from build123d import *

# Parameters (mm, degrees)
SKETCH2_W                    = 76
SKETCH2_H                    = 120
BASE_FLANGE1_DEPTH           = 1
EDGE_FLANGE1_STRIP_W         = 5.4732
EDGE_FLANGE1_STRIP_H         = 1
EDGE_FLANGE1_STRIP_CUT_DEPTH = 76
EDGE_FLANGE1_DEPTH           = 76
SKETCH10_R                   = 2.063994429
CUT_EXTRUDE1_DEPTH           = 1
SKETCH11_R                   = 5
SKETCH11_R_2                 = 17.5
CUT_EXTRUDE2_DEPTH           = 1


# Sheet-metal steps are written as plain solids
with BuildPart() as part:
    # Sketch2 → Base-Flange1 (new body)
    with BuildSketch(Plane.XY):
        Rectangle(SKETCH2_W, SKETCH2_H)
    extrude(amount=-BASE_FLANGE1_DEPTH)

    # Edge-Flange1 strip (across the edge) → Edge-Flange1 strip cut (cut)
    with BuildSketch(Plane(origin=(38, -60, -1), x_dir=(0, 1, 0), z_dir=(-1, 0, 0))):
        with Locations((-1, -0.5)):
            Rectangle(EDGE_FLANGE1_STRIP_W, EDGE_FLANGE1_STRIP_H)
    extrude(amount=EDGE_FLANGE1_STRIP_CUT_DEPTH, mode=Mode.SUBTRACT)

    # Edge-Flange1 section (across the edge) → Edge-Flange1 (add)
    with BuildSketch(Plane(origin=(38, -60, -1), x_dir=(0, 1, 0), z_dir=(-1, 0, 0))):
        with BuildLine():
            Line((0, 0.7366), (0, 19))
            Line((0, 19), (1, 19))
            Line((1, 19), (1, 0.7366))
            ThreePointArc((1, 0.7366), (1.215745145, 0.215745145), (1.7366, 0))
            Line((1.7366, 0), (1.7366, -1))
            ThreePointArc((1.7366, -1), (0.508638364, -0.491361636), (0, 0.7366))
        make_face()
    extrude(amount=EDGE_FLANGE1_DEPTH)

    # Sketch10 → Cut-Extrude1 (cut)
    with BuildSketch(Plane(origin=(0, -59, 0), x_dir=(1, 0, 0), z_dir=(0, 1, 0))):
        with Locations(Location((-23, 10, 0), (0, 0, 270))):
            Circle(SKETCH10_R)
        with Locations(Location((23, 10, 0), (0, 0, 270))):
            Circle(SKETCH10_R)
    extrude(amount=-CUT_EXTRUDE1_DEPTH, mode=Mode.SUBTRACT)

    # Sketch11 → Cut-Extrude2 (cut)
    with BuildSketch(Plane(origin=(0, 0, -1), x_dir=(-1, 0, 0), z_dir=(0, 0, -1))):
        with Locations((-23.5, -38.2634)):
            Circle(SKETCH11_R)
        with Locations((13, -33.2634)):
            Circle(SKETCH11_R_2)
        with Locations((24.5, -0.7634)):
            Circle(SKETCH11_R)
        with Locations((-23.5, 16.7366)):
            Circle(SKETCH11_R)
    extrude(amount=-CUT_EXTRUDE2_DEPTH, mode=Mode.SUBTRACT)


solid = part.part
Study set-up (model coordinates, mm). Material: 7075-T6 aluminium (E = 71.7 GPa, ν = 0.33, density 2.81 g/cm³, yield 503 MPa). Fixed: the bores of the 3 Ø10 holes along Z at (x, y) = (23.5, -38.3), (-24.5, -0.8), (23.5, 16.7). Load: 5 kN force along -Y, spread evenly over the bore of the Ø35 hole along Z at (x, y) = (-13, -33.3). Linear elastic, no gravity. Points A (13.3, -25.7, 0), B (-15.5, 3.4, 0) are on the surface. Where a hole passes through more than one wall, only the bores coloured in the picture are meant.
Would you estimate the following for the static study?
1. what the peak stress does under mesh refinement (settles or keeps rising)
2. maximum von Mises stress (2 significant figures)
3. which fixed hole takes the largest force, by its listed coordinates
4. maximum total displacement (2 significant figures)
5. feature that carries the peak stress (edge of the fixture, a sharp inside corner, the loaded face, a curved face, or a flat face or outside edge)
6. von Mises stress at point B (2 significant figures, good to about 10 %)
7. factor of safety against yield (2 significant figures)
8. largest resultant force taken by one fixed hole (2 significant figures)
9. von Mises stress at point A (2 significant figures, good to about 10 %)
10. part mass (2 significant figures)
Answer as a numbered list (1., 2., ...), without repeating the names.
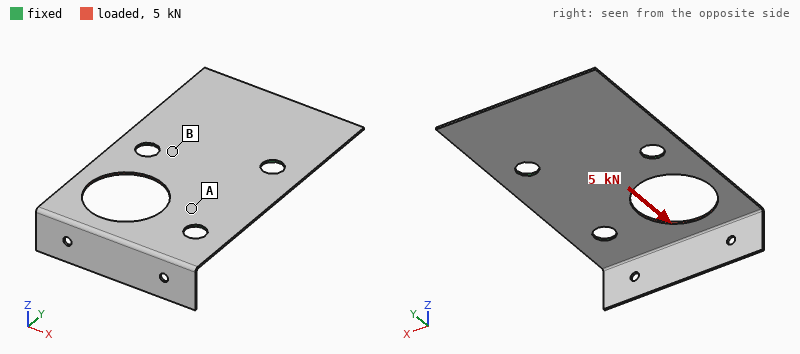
1. settles
2. 360 MPa
3. (-24.5, -0.8)
4. 0.17 mm
5. the loaded face
6. 28 MPa
7. 1.4
8. 2.9 kN
9. 73 MPa
10. 26 g
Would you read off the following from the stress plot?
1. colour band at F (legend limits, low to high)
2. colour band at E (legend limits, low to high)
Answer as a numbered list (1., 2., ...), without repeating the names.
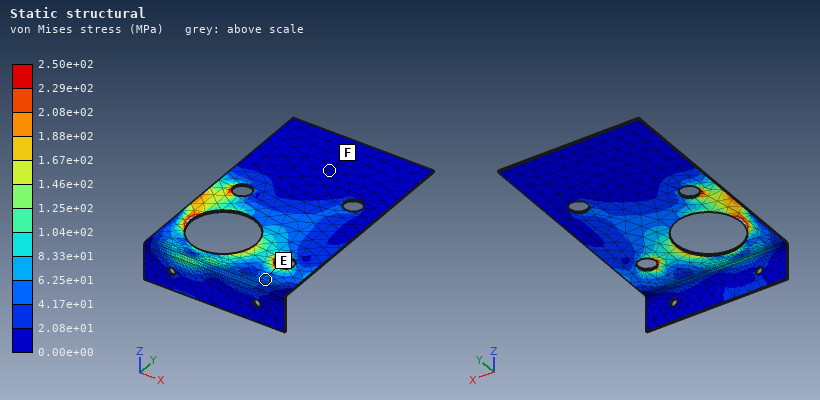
1. 0.00e+00 to 2.08e+01 MPa
2. 4.17e+01 to 6.25e+01 MPa
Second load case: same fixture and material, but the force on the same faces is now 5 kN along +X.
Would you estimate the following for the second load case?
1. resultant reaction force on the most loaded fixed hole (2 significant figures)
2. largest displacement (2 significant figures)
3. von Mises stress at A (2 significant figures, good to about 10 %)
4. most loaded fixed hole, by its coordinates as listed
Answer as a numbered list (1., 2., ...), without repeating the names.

1. 3.2 kN
2. 0.20 mm
3. 62 MPa
4. (23.5, -38.3)
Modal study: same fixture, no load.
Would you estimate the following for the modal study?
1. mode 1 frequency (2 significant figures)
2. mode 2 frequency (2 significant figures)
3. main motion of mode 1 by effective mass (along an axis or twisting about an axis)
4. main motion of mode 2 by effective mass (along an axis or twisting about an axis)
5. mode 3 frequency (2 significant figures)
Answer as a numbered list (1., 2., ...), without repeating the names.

1. 330 Hz
2. 350 Hz
3. along Z
4. along Z
5. 690 Hz
